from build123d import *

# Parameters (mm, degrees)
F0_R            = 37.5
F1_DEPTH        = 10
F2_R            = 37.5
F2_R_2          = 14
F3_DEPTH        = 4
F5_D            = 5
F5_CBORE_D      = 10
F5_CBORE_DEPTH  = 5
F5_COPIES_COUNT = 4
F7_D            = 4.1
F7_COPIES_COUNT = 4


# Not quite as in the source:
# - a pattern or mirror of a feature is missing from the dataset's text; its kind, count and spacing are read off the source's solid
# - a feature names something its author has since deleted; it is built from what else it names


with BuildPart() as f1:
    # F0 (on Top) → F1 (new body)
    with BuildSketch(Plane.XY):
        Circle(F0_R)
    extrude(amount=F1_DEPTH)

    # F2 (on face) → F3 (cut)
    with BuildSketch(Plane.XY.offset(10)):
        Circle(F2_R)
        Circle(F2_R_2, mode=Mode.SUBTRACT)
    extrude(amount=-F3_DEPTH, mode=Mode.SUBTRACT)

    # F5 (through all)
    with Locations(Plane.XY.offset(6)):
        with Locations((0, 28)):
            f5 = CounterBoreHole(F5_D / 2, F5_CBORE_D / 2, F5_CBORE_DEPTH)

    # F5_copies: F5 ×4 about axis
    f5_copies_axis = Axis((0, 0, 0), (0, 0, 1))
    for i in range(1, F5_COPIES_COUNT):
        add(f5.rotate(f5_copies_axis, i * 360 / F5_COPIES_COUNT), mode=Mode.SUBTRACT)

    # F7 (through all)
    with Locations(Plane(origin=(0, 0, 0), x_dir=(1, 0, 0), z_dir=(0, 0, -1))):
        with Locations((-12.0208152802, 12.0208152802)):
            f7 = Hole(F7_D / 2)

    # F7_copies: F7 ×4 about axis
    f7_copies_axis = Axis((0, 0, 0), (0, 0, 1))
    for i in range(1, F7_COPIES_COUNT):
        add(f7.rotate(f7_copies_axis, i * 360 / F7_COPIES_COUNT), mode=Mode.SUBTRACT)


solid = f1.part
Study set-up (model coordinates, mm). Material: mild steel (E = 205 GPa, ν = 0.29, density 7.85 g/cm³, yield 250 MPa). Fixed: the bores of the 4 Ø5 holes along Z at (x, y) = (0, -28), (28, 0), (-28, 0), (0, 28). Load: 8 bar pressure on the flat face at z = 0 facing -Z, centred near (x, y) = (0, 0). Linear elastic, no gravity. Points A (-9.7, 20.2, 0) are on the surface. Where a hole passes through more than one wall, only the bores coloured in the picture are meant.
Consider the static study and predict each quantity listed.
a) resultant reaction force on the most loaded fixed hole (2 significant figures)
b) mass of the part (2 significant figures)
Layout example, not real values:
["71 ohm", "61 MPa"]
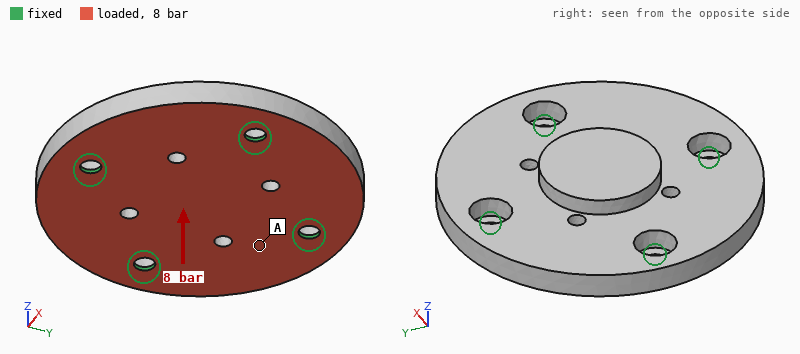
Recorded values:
["900 N", "210 g"]
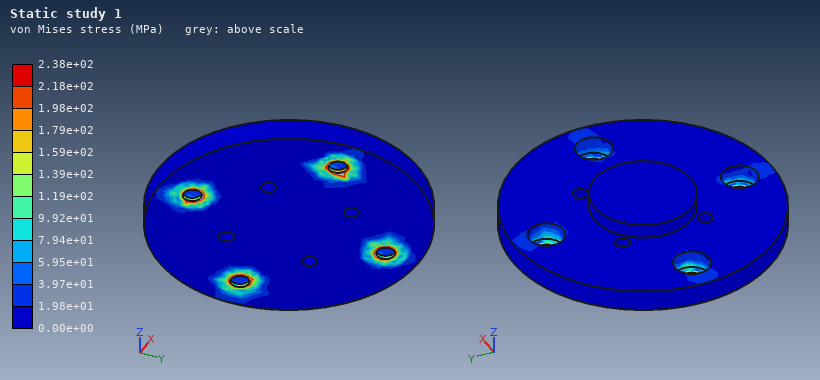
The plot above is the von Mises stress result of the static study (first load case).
